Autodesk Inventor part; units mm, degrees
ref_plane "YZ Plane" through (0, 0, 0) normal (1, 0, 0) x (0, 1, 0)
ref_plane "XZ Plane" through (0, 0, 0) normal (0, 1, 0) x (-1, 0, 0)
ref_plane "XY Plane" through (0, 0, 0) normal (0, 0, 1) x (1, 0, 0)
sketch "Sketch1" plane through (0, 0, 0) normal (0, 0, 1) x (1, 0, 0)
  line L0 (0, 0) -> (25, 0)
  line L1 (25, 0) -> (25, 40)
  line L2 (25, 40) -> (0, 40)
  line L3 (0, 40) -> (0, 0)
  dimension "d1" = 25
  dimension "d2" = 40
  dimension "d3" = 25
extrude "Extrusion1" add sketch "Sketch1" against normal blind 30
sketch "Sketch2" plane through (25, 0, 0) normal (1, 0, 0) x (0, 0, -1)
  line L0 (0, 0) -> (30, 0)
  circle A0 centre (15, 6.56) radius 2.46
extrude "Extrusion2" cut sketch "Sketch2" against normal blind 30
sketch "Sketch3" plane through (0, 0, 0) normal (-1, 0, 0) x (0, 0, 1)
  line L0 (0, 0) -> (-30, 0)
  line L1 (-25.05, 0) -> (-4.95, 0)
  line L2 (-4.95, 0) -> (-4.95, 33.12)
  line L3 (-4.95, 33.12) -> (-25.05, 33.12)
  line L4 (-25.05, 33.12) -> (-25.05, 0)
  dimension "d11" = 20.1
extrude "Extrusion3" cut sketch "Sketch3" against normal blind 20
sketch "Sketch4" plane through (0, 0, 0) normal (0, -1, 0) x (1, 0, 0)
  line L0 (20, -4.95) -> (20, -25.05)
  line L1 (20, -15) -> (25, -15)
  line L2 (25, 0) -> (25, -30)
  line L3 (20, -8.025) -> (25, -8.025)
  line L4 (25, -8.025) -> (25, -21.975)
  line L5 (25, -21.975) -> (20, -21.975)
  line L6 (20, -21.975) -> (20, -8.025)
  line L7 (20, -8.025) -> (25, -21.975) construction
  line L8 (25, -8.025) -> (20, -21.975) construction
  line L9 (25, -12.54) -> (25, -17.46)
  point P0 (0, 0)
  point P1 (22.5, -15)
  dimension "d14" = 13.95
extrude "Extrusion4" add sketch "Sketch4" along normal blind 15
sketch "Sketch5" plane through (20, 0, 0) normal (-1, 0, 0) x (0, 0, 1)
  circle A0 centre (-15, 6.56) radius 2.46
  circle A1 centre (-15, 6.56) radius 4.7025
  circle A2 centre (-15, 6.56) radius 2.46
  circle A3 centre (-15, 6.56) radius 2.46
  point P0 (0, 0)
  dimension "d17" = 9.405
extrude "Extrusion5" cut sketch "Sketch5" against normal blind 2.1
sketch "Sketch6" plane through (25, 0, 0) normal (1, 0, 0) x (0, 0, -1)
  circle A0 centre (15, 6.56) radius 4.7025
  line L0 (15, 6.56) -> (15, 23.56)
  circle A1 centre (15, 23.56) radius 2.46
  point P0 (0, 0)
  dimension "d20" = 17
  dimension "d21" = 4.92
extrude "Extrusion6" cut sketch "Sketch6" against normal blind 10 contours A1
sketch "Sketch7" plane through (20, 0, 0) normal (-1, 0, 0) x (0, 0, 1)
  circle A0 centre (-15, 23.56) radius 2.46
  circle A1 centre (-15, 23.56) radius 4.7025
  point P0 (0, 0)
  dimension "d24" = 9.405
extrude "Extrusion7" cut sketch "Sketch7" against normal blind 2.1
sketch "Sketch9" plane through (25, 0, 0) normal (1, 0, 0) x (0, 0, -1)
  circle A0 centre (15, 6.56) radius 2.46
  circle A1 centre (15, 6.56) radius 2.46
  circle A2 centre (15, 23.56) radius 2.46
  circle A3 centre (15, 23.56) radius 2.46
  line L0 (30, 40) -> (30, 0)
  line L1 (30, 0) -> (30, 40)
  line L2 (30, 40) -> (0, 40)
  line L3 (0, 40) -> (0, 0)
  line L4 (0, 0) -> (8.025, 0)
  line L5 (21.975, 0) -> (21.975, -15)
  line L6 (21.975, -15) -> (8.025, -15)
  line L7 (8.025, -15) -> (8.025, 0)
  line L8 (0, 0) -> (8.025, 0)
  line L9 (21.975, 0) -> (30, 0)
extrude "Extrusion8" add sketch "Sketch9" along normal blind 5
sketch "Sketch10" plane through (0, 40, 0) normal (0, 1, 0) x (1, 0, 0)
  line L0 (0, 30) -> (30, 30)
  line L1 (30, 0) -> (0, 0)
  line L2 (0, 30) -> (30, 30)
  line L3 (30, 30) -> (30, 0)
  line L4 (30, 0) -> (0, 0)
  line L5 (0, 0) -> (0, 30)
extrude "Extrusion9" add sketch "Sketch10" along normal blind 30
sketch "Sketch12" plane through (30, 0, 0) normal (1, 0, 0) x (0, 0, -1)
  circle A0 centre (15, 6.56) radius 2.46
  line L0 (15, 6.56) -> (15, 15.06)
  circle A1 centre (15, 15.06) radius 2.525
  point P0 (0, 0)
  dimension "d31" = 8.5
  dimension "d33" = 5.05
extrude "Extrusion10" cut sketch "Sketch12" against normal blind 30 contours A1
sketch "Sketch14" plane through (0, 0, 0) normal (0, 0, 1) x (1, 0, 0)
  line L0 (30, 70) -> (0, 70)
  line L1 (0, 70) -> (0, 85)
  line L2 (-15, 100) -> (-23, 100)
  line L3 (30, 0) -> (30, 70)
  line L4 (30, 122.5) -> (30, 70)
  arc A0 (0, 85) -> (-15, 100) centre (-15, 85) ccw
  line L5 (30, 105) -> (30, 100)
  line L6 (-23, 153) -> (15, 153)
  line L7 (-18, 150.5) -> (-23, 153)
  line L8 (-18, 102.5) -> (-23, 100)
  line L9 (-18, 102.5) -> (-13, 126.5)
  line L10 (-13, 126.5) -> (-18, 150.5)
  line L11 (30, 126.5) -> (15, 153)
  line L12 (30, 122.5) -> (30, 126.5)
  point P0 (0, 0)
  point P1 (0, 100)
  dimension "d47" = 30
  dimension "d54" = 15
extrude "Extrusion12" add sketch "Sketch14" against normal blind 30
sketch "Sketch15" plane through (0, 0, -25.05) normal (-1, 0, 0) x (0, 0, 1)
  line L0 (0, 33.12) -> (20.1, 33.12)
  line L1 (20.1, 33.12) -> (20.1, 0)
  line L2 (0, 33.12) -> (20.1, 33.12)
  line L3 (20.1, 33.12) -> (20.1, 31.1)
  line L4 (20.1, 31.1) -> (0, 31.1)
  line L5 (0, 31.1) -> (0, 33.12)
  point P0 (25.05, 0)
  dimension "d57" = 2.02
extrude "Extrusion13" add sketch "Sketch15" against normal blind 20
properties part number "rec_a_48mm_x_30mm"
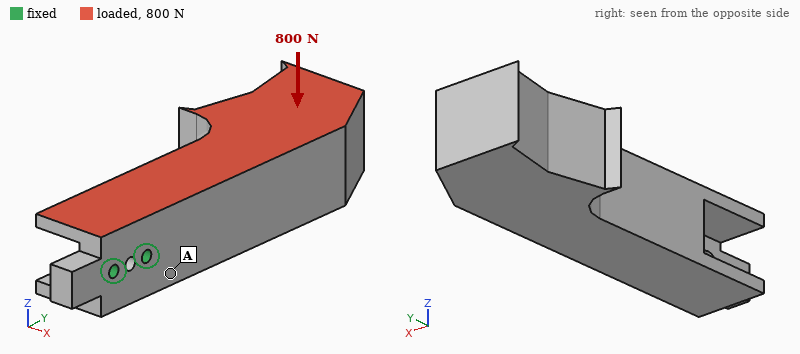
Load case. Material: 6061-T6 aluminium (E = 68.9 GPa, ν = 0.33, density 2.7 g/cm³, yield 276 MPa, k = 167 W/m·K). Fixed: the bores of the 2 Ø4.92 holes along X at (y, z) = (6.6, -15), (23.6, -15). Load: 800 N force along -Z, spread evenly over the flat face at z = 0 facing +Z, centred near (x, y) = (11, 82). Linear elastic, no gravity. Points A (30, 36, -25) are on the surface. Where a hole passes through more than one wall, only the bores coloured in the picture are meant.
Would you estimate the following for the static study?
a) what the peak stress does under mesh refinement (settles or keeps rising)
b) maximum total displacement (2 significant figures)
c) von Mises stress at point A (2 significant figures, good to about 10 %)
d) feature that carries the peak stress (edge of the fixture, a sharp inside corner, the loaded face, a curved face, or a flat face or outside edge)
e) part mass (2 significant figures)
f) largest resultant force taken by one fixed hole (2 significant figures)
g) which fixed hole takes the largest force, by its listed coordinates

keeps rising
0.15 mm
8.9 MPa
edge of the fixture
400 g
2.8 kN
(23.6, -15)
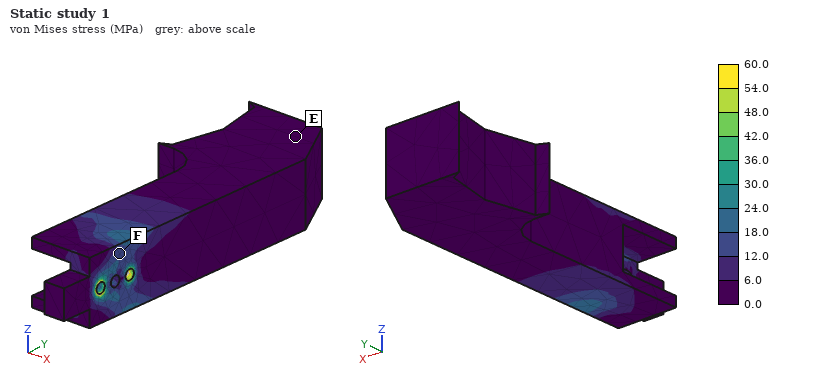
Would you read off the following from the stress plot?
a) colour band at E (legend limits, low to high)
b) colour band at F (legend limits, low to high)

0.0 to 6.0 MPa
12.0 to 18.0 MPa
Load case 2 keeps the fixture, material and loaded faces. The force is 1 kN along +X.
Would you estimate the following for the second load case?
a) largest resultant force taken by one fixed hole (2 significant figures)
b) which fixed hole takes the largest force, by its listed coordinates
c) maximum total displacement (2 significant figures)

3.3 kN
(23.6, -15)
0.25 mm
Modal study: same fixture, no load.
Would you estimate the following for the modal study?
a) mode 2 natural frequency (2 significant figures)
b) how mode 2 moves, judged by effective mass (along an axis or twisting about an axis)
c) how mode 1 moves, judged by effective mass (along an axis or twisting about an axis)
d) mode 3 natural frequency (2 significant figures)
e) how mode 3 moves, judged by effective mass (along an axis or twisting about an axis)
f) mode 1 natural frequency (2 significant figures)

720 Hz
along Z
along X
2300 Hz
twisting about Y
610 Hz
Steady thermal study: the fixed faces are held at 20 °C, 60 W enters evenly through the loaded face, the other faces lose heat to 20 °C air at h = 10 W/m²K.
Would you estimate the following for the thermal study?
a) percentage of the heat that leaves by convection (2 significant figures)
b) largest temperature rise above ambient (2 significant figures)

6.4 %
31 K
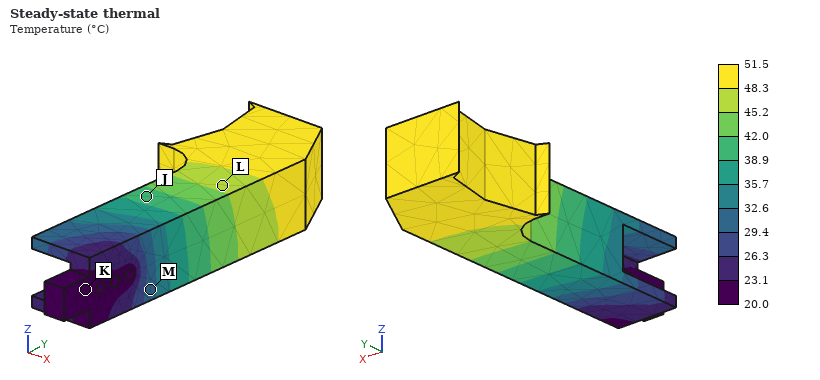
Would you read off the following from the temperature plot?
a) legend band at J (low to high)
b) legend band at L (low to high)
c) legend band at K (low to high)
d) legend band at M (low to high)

38.9 to 42.0 °C
45.2 to 48.3 °C
20.0 to 23.1 °C
29.4 to 32.6 °C
